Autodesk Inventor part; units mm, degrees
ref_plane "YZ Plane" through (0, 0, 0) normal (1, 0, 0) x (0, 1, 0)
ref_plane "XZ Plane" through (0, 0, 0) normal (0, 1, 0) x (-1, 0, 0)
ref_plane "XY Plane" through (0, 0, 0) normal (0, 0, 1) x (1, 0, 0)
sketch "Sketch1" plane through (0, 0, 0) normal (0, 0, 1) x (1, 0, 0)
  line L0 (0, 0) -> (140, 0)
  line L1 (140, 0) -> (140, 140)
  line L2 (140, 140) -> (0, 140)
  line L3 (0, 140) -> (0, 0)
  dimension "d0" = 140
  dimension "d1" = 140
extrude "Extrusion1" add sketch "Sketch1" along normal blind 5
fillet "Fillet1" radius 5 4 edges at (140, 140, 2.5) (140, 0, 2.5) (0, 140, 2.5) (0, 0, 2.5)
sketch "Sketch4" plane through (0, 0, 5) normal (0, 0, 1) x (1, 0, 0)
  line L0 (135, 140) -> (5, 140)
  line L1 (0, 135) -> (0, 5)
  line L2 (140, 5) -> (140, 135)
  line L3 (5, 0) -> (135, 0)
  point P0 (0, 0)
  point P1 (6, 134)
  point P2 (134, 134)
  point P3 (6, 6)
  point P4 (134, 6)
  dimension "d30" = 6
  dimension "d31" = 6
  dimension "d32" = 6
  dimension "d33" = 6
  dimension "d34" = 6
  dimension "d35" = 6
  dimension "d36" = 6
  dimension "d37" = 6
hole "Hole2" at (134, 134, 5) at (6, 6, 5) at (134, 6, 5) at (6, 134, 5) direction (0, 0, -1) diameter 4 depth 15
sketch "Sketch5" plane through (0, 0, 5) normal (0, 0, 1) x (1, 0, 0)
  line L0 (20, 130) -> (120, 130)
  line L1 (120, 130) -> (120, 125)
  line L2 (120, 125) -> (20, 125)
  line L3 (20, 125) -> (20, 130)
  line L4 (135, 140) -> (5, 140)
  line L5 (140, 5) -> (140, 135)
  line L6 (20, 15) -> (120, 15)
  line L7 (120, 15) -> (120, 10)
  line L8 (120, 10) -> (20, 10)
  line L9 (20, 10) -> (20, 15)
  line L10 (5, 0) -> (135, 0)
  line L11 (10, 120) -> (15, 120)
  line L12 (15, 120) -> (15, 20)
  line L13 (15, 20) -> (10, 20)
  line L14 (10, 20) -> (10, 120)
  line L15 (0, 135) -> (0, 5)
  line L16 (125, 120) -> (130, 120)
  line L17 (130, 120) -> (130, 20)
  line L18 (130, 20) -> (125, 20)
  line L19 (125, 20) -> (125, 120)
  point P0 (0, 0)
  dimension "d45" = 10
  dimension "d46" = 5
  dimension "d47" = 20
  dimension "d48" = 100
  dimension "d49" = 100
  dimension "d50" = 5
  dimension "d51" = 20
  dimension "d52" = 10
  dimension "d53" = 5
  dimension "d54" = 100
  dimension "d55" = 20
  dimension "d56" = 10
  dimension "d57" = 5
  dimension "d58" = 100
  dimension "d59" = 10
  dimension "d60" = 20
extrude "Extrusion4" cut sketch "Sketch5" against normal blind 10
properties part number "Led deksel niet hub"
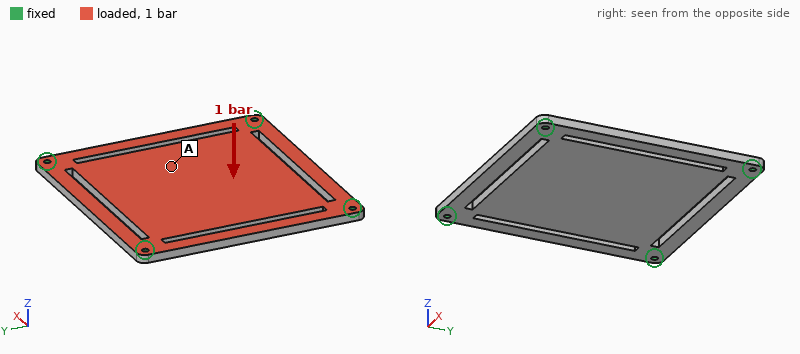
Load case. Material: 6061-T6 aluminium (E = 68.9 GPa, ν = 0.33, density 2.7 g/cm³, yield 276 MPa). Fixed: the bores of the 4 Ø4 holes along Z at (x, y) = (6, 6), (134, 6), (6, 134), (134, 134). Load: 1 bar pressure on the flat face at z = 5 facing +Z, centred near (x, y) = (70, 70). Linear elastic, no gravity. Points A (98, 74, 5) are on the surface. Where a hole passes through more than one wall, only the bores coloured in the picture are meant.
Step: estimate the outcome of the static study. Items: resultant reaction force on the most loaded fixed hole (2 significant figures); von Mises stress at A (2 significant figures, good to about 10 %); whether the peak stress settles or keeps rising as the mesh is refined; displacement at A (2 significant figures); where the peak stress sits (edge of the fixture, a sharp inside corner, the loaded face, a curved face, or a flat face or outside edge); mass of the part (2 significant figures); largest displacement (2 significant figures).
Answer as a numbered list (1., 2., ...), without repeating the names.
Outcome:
1. 440 N
2. 24 MPa
3. keeps rising
4. 0.32 mm
5. edge of the fixture
6. 240 g
7. 0.36 mm
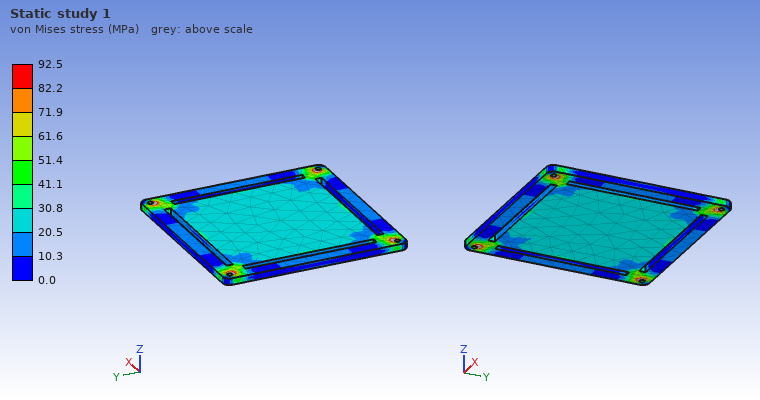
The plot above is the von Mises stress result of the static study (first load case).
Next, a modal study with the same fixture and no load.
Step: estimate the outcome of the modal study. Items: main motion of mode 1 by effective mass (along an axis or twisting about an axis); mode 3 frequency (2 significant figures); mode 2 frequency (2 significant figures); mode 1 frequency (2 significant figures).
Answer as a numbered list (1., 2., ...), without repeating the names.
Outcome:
1. along Z
2. 1600 Hz
3. 1600 Hz
4. 830 Hz
